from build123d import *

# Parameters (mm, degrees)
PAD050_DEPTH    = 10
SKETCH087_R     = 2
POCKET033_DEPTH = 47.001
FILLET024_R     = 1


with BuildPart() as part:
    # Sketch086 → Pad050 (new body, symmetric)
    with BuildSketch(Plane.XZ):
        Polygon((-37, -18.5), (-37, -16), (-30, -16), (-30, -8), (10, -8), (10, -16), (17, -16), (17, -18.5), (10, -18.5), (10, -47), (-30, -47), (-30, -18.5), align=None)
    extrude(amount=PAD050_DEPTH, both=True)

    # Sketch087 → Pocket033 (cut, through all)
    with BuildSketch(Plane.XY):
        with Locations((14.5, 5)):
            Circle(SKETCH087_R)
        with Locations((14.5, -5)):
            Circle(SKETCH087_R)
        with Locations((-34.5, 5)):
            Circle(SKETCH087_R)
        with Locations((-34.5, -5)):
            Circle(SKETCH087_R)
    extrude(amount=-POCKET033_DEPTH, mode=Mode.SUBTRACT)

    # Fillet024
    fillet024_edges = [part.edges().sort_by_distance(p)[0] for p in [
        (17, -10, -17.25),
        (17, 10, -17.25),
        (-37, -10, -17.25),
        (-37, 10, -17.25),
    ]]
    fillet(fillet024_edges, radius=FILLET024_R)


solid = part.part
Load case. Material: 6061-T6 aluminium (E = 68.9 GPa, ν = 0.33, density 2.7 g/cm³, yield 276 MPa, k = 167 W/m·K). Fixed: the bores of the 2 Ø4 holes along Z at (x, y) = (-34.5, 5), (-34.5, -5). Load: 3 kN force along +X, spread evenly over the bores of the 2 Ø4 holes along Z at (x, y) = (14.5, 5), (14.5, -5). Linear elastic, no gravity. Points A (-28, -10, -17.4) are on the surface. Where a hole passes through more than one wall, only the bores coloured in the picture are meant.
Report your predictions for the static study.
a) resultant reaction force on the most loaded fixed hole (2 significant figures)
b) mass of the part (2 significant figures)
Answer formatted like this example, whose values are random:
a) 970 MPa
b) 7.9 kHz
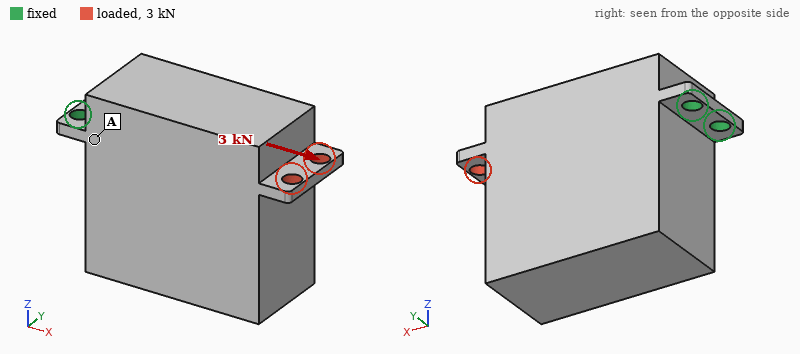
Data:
a) 1.5 kN
b) 86 g
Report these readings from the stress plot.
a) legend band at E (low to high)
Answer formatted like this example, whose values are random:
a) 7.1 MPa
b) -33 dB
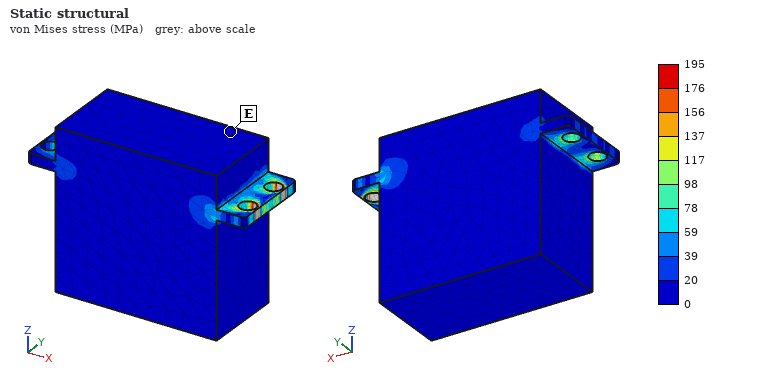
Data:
a) 0 to 20 MPa
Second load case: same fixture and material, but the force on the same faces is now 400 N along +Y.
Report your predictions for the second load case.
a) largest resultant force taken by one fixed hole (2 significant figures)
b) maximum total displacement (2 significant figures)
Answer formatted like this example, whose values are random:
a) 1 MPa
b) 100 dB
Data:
a) 1.6 kN
b) 79 µm
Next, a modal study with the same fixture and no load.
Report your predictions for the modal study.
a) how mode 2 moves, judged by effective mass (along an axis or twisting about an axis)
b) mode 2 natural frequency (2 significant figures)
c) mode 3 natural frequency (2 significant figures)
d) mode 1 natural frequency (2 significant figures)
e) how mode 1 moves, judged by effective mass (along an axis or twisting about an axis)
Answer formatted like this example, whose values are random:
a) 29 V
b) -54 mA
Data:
a) along Y
b) 1800 Hz
c) 3400 Hz
d) 410 Hz
e) along Z
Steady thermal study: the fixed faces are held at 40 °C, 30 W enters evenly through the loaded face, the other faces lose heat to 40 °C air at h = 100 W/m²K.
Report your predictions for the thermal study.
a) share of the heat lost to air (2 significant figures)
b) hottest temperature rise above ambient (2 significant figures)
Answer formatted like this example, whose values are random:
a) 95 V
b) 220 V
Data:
a) 37 %
b) 56 K
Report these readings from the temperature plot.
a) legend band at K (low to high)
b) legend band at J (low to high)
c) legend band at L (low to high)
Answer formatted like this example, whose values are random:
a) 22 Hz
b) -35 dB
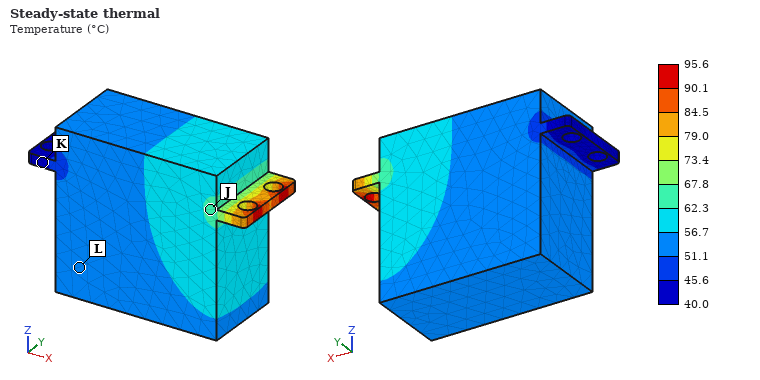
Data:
a) 40.0 to 45.6 °C
b) 62.3 to 67.8 °C
c) 51.1 to 56.7 °C
